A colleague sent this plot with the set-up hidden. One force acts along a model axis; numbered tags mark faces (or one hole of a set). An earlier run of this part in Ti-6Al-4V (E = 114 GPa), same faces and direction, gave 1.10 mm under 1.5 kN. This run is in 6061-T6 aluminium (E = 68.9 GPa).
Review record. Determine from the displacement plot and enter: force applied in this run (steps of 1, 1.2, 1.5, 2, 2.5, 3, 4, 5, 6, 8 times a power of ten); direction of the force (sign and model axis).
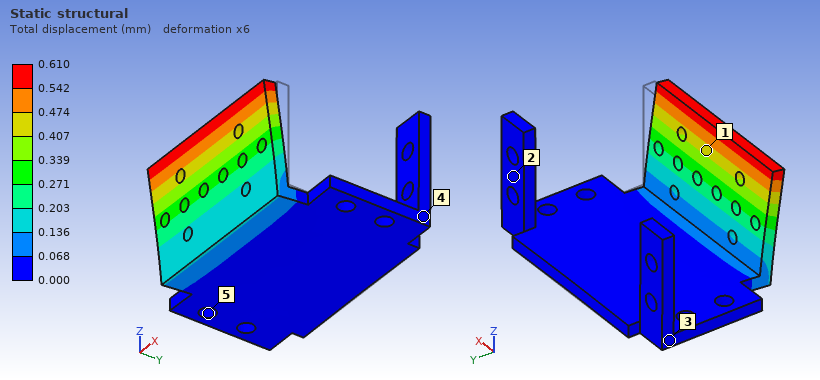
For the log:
500 N
-Y
